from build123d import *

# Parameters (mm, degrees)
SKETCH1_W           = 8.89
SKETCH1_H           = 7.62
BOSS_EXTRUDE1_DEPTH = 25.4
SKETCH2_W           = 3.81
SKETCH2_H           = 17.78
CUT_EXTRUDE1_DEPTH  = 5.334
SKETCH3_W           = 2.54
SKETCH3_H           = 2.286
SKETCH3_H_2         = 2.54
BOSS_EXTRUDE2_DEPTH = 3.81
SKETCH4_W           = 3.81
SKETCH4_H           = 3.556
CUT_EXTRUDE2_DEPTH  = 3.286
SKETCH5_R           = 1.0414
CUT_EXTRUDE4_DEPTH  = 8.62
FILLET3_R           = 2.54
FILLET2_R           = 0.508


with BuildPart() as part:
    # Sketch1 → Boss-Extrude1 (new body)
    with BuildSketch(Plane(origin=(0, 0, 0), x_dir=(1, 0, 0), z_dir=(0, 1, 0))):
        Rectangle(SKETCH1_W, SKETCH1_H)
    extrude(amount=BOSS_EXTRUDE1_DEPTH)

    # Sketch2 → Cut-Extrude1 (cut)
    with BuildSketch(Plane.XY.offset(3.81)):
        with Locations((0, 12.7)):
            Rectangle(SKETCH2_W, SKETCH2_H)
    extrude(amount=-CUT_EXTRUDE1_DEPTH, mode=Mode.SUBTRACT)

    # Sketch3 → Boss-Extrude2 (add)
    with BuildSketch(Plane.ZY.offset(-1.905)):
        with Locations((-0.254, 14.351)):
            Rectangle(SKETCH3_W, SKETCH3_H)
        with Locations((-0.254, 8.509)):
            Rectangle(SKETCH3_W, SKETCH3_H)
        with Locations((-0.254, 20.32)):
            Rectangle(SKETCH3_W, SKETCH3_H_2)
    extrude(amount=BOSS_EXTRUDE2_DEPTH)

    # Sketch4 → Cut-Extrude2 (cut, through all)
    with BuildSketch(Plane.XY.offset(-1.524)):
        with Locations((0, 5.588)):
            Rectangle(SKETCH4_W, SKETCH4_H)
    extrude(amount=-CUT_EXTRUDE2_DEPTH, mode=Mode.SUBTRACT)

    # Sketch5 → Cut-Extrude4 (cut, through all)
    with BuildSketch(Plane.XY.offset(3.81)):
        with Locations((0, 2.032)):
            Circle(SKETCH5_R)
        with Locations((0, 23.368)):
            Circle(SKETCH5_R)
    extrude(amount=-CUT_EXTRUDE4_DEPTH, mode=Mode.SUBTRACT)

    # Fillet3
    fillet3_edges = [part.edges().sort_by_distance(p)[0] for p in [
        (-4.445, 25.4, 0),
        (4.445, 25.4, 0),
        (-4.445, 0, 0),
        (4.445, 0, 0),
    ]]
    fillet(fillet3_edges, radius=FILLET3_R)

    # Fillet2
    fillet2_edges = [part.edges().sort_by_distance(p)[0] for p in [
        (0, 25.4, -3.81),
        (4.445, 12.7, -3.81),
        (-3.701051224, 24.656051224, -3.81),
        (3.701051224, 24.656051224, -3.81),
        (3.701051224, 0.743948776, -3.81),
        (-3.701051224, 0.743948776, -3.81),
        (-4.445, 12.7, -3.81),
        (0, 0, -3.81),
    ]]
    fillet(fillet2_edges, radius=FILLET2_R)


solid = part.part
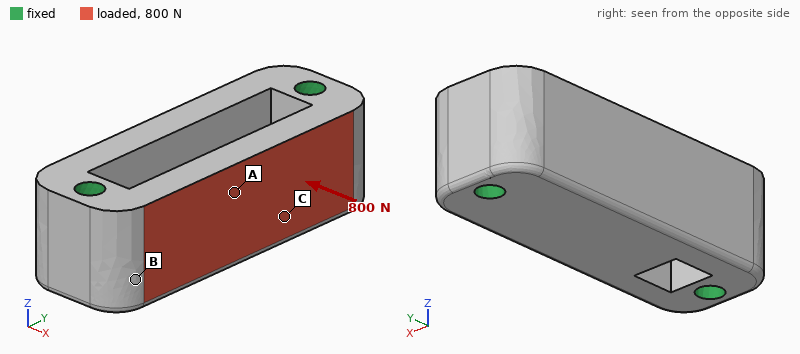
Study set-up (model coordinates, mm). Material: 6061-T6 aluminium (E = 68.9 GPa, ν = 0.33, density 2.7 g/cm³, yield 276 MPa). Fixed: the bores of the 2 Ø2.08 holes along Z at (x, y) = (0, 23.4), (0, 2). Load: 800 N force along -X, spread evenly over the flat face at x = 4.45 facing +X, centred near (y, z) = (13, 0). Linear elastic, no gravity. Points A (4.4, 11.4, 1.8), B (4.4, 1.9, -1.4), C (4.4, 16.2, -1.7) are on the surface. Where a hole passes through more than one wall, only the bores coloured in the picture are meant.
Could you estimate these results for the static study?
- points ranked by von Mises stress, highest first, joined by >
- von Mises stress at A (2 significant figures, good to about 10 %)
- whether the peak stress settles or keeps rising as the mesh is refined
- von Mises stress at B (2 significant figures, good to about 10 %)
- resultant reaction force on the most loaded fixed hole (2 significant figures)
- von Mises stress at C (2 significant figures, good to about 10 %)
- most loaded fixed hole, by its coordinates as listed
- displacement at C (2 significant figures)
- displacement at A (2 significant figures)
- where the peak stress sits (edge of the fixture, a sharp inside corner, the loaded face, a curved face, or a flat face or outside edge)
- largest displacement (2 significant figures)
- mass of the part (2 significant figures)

A > C > B
31 MPa
keeps rising
11 MPa
430 N
23 MPa
(0, 23.4)
5.7 µm
9.9 µm
edge of the fixture
12 µm
3.5 g
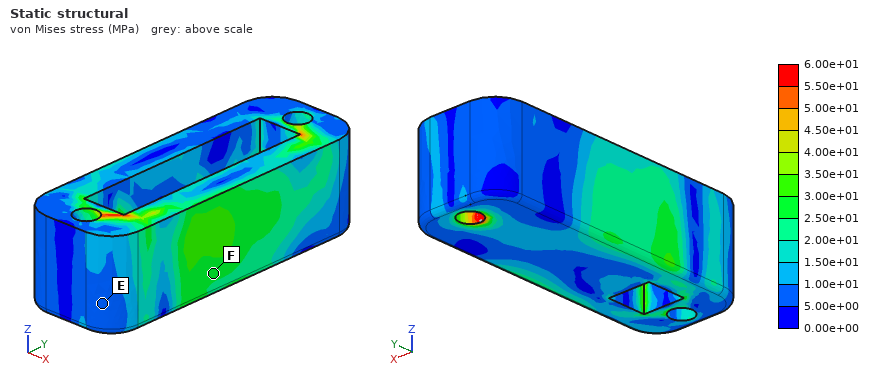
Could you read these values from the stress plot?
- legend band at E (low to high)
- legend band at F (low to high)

5.00e+00 to 1.00e+01 MPa
2.50e+01 to 3.00e+01 MPa
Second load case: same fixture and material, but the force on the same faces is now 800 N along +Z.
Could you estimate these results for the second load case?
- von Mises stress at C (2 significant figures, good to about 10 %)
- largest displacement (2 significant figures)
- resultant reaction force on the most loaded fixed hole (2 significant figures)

29 MPa
14 µm
420 N
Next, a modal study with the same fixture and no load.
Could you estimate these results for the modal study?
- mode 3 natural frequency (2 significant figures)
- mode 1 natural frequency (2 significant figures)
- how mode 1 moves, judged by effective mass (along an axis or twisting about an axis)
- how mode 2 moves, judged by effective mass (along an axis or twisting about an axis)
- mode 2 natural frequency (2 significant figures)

52 kHz
35 kHz
along X
along Z
44 kHz
